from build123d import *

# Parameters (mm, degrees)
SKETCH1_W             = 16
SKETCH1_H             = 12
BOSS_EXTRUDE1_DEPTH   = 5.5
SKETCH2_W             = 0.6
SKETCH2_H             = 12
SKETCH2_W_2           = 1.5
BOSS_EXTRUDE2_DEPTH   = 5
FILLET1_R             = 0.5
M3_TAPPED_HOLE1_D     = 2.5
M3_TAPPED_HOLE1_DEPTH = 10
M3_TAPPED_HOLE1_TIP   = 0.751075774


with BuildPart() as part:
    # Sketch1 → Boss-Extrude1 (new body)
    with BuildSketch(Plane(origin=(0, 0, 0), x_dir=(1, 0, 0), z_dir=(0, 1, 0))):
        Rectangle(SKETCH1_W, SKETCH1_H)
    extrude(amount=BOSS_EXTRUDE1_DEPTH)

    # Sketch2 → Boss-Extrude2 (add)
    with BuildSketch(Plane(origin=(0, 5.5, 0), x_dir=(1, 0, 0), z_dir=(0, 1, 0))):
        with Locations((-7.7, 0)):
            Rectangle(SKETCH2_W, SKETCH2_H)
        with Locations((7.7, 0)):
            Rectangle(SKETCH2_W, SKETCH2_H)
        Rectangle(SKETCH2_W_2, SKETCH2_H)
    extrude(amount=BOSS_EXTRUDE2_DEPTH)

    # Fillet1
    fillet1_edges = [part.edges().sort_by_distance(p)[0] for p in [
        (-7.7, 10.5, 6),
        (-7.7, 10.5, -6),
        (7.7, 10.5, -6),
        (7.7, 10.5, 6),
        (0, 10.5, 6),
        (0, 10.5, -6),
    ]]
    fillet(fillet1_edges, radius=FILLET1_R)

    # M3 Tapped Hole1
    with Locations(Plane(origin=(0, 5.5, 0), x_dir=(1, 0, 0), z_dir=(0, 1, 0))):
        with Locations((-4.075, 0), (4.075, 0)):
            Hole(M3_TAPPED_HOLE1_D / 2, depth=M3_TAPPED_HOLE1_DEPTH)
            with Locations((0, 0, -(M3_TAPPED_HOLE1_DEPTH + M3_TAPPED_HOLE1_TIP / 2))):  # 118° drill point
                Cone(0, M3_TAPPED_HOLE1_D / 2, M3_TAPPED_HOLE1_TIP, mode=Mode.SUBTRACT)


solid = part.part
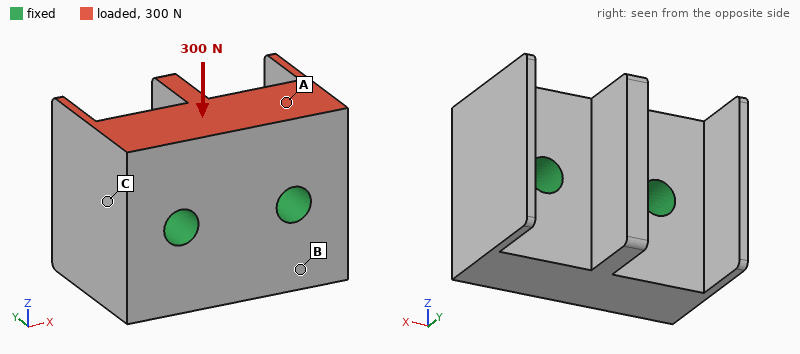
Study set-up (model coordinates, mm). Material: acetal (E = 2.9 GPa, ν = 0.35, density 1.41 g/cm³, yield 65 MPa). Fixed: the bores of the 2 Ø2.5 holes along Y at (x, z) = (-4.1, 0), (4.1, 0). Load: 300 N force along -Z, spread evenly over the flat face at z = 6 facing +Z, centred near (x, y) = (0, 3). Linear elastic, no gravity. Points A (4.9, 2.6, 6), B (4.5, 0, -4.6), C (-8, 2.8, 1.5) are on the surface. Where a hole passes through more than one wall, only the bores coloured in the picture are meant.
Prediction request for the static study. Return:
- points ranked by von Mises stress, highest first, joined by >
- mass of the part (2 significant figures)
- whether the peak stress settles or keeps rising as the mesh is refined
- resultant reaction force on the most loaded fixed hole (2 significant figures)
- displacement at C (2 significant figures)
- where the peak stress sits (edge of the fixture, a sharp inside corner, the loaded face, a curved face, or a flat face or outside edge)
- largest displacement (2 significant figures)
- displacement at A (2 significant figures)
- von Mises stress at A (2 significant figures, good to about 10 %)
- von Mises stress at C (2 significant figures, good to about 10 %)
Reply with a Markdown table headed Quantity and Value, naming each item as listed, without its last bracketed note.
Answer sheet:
| Quantity | Value |
|---|---|
| points ranked by von Mises stress, highest first, joined by > | A > C > B |
| mass of the part | 1.6 g |
| whether the peak stress settles or keeps rising as the mesh is refined | keeps rising |
| resultant reaction force on the most loaded fixed hole | 150 N |
| displacement at C | 5.0 µm |
| where the peak stress sits | edge of the fixture |
| largest displacement | 17 µm |
| displacement at A | 7.5 µm |
| von Mises stress at A | 3.7 MPa |
| von Mises stress at C | 1.9 MPa |
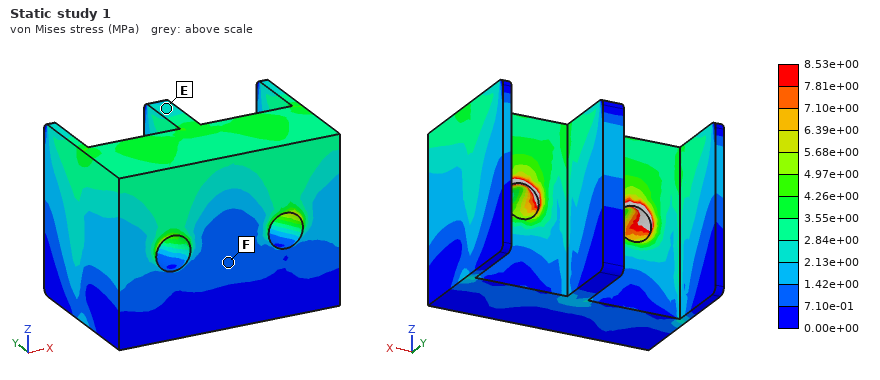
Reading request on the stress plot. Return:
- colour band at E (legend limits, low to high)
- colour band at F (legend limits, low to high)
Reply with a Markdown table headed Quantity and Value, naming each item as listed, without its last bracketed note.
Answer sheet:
| Quantity | Value |
|---|---|
| colour band at E | 2.13e+00 to 2.84e+00 MPa |
| colour band at F | 7.10e-01 to 1.42e+00 MPa |
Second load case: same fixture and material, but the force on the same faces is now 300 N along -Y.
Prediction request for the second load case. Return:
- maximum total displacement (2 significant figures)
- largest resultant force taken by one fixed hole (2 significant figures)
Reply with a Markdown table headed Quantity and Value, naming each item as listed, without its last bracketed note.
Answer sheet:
| Quantity | Value |
|---|---|
| maximum total displacement | 67 µm |
| largest resultant force taken by one fixed hole | 150 N |
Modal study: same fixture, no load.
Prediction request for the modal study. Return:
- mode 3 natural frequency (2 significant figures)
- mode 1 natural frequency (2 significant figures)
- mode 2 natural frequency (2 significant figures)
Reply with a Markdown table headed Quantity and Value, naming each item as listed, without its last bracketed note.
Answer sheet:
| Quantity | Value |
|---|---|
| mode 3 natural frequency | 7100 Hz |
| mode 1 natural frequency | 5100 Hz |
| mode 2 natural frequency | 5100 Hz |
